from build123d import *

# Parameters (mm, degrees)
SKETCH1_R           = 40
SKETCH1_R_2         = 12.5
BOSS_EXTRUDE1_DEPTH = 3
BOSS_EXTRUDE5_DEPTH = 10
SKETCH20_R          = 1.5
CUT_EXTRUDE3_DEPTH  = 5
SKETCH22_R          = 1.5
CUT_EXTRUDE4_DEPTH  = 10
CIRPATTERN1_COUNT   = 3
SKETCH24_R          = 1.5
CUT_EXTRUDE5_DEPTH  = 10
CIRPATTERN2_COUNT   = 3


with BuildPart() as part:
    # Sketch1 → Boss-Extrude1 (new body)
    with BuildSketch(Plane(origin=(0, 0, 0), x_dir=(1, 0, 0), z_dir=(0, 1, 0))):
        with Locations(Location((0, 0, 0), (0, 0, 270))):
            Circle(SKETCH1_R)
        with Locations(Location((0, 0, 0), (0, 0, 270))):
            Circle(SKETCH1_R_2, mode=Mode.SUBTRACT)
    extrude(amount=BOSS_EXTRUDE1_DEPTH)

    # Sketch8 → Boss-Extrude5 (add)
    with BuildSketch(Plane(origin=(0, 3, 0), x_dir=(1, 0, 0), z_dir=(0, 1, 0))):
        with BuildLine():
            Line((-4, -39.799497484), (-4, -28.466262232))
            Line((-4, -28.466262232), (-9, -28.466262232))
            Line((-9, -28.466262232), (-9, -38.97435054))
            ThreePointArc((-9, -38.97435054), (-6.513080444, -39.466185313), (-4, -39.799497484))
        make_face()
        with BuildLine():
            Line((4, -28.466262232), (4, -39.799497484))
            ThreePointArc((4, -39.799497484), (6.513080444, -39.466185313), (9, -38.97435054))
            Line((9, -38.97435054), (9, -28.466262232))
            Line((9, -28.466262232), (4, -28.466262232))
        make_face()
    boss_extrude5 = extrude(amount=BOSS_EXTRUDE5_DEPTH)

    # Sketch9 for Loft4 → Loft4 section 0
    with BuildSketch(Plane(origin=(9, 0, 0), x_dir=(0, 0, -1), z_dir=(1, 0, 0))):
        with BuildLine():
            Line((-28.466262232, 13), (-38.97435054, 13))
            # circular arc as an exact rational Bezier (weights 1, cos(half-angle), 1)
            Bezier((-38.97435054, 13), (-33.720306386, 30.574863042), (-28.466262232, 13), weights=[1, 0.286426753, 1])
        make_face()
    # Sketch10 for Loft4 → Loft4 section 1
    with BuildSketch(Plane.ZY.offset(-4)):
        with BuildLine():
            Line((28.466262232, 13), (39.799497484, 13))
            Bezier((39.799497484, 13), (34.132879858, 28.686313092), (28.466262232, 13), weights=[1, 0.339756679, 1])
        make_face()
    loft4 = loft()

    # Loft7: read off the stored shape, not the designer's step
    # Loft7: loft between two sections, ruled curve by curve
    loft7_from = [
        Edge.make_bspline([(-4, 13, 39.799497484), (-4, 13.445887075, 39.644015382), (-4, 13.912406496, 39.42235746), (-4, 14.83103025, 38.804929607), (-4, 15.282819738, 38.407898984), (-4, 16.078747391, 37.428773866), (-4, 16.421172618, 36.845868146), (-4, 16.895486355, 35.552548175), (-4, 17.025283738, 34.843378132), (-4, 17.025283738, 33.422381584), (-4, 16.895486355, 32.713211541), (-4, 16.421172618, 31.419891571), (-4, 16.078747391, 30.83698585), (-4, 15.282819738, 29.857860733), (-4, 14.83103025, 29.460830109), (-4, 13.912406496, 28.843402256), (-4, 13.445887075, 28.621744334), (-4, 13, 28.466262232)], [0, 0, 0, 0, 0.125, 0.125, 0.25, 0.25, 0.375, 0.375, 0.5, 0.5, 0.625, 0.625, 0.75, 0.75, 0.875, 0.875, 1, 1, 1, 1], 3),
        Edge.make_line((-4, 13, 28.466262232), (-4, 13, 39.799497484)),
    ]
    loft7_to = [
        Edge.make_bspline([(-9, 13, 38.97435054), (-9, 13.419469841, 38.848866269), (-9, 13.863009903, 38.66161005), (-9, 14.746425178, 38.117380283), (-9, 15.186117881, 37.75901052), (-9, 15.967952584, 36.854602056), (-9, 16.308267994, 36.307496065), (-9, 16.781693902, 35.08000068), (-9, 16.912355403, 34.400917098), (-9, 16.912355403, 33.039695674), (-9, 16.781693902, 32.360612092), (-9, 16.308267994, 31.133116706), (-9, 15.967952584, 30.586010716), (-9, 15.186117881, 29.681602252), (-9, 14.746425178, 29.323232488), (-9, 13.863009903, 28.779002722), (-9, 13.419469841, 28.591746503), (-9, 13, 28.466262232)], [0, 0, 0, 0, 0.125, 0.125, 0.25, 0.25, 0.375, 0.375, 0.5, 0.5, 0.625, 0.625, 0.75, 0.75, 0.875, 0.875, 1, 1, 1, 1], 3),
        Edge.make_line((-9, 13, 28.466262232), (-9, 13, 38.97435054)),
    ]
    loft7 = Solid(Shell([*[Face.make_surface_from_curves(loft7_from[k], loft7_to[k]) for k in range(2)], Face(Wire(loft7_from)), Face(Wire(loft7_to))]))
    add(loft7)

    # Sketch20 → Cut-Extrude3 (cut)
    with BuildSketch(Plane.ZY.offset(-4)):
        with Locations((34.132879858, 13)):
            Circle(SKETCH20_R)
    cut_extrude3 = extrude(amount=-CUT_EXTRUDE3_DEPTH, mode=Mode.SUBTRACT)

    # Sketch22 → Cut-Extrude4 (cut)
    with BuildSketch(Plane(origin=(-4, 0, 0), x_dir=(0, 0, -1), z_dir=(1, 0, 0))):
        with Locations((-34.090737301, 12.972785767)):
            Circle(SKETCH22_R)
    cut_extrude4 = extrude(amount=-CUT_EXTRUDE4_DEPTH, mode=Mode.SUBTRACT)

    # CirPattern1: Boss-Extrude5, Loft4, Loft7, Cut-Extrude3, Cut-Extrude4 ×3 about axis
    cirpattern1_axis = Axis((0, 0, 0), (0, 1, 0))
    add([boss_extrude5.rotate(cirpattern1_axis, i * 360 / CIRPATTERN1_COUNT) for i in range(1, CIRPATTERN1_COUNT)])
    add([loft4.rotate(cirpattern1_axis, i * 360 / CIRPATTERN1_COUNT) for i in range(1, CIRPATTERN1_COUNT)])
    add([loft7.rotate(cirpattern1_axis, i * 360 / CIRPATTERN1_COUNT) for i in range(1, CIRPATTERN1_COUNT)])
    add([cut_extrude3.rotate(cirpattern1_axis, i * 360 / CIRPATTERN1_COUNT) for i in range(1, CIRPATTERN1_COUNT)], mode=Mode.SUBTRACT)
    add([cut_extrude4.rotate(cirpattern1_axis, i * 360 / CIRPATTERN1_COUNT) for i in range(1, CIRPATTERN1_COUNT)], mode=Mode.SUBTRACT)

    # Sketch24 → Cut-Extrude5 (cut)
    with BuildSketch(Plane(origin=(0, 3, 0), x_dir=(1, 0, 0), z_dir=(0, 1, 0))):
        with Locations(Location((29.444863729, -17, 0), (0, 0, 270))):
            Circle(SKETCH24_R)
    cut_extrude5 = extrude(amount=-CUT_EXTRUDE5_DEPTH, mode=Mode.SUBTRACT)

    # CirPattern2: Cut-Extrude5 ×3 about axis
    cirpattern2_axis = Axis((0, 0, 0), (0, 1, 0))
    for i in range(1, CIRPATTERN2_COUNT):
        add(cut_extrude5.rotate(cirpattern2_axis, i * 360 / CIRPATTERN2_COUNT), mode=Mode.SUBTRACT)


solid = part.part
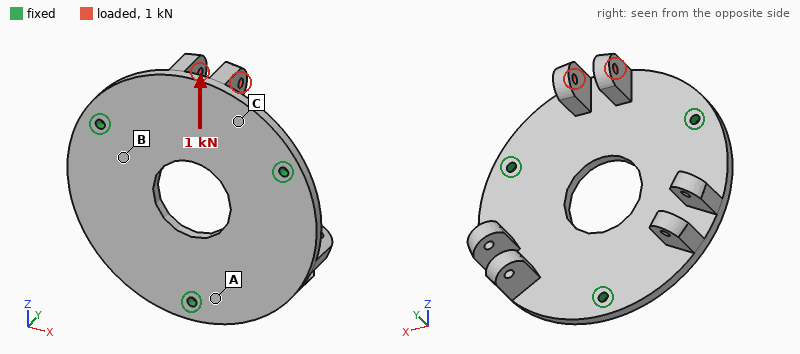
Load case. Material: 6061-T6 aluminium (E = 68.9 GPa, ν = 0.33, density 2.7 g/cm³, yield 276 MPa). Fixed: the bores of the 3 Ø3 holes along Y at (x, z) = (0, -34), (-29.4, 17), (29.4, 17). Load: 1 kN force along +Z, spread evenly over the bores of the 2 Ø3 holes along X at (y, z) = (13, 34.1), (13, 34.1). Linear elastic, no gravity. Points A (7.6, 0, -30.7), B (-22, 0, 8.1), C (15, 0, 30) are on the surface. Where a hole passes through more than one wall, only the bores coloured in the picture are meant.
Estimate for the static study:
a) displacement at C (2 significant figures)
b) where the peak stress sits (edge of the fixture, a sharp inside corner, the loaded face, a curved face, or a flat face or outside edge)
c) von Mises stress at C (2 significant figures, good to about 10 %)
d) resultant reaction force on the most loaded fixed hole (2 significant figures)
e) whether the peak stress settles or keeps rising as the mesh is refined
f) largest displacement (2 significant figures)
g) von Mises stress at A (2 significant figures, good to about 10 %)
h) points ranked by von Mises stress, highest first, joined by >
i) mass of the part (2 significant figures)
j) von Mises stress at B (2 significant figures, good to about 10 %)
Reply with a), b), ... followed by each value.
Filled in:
a) 0.22 mm
b) edge of the fixture
c) 140 MPa
d) 480 N
e) keeps rising
f) 0.69 mm
g) 17 MPa
h) C > B > A
i) 47 g
j) 34 MPa
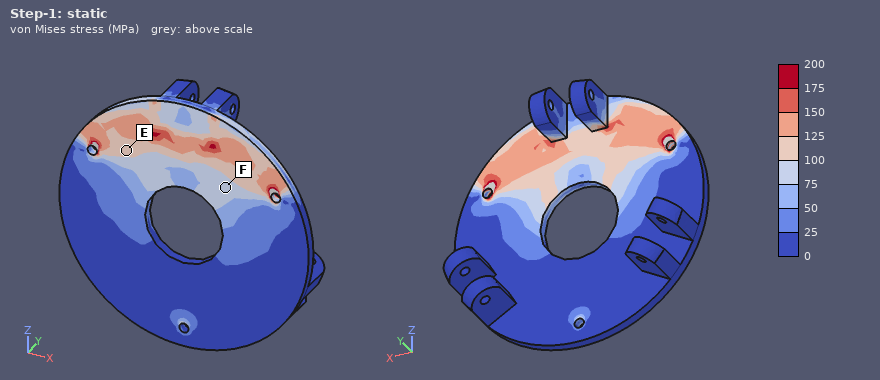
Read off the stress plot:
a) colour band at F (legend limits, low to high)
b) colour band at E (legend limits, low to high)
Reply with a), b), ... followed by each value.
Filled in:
a) 75 to 100 MPa
b) 100 to 125 MPa
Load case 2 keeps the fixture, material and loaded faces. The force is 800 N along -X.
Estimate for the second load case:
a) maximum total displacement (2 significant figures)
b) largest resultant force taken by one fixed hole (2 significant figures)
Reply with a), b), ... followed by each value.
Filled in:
a) 0.17 mm
b) 500 N
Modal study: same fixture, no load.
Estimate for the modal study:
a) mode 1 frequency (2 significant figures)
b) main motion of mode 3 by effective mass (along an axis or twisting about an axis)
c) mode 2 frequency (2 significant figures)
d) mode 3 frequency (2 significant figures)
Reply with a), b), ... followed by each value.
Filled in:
a) 2000 Hz
b) along Y
c) 2000 Hz
d) 2400 Hz
